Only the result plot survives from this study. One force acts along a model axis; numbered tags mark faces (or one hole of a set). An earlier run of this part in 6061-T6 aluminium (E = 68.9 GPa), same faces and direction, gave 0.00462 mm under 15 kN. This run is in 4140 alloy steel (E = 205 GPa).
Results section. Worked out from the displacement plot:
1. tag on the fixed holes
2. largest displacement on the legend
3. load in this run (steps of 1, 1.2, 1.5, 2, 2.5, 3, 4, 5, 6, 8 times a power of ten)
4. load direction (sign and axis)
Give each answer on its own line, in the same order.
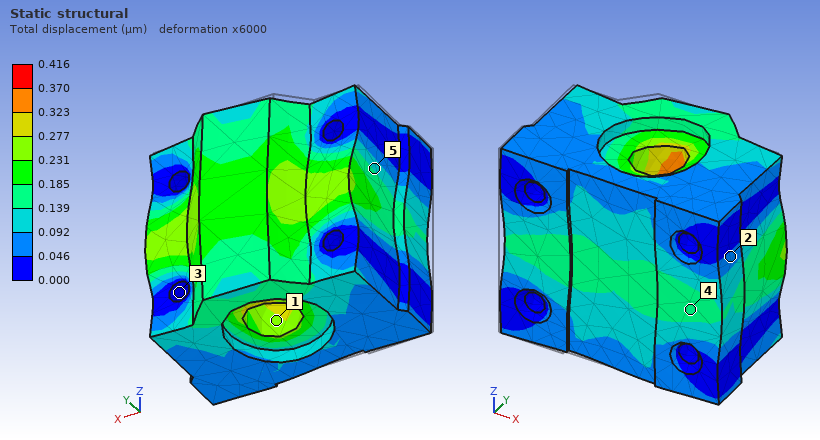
3
0.416 µm
4 kN
+X
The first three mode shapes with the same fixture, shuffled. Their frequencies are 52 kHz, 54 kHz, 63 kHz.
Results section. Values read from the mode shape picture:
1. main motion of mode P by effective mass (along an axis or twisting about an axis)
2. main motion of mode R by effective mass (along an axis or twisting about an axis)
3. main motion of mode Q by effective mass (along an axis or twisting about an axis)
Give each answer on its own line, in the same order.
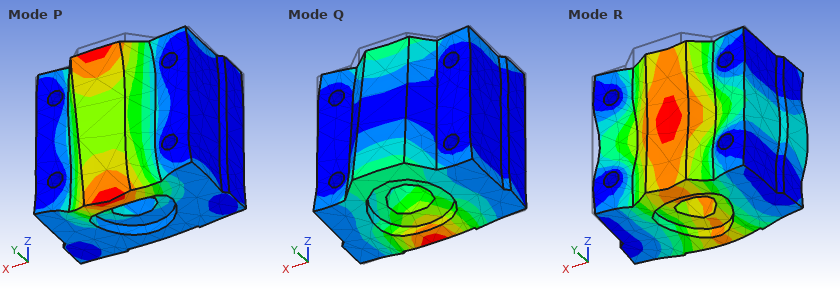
along Z
along Y
along Z
